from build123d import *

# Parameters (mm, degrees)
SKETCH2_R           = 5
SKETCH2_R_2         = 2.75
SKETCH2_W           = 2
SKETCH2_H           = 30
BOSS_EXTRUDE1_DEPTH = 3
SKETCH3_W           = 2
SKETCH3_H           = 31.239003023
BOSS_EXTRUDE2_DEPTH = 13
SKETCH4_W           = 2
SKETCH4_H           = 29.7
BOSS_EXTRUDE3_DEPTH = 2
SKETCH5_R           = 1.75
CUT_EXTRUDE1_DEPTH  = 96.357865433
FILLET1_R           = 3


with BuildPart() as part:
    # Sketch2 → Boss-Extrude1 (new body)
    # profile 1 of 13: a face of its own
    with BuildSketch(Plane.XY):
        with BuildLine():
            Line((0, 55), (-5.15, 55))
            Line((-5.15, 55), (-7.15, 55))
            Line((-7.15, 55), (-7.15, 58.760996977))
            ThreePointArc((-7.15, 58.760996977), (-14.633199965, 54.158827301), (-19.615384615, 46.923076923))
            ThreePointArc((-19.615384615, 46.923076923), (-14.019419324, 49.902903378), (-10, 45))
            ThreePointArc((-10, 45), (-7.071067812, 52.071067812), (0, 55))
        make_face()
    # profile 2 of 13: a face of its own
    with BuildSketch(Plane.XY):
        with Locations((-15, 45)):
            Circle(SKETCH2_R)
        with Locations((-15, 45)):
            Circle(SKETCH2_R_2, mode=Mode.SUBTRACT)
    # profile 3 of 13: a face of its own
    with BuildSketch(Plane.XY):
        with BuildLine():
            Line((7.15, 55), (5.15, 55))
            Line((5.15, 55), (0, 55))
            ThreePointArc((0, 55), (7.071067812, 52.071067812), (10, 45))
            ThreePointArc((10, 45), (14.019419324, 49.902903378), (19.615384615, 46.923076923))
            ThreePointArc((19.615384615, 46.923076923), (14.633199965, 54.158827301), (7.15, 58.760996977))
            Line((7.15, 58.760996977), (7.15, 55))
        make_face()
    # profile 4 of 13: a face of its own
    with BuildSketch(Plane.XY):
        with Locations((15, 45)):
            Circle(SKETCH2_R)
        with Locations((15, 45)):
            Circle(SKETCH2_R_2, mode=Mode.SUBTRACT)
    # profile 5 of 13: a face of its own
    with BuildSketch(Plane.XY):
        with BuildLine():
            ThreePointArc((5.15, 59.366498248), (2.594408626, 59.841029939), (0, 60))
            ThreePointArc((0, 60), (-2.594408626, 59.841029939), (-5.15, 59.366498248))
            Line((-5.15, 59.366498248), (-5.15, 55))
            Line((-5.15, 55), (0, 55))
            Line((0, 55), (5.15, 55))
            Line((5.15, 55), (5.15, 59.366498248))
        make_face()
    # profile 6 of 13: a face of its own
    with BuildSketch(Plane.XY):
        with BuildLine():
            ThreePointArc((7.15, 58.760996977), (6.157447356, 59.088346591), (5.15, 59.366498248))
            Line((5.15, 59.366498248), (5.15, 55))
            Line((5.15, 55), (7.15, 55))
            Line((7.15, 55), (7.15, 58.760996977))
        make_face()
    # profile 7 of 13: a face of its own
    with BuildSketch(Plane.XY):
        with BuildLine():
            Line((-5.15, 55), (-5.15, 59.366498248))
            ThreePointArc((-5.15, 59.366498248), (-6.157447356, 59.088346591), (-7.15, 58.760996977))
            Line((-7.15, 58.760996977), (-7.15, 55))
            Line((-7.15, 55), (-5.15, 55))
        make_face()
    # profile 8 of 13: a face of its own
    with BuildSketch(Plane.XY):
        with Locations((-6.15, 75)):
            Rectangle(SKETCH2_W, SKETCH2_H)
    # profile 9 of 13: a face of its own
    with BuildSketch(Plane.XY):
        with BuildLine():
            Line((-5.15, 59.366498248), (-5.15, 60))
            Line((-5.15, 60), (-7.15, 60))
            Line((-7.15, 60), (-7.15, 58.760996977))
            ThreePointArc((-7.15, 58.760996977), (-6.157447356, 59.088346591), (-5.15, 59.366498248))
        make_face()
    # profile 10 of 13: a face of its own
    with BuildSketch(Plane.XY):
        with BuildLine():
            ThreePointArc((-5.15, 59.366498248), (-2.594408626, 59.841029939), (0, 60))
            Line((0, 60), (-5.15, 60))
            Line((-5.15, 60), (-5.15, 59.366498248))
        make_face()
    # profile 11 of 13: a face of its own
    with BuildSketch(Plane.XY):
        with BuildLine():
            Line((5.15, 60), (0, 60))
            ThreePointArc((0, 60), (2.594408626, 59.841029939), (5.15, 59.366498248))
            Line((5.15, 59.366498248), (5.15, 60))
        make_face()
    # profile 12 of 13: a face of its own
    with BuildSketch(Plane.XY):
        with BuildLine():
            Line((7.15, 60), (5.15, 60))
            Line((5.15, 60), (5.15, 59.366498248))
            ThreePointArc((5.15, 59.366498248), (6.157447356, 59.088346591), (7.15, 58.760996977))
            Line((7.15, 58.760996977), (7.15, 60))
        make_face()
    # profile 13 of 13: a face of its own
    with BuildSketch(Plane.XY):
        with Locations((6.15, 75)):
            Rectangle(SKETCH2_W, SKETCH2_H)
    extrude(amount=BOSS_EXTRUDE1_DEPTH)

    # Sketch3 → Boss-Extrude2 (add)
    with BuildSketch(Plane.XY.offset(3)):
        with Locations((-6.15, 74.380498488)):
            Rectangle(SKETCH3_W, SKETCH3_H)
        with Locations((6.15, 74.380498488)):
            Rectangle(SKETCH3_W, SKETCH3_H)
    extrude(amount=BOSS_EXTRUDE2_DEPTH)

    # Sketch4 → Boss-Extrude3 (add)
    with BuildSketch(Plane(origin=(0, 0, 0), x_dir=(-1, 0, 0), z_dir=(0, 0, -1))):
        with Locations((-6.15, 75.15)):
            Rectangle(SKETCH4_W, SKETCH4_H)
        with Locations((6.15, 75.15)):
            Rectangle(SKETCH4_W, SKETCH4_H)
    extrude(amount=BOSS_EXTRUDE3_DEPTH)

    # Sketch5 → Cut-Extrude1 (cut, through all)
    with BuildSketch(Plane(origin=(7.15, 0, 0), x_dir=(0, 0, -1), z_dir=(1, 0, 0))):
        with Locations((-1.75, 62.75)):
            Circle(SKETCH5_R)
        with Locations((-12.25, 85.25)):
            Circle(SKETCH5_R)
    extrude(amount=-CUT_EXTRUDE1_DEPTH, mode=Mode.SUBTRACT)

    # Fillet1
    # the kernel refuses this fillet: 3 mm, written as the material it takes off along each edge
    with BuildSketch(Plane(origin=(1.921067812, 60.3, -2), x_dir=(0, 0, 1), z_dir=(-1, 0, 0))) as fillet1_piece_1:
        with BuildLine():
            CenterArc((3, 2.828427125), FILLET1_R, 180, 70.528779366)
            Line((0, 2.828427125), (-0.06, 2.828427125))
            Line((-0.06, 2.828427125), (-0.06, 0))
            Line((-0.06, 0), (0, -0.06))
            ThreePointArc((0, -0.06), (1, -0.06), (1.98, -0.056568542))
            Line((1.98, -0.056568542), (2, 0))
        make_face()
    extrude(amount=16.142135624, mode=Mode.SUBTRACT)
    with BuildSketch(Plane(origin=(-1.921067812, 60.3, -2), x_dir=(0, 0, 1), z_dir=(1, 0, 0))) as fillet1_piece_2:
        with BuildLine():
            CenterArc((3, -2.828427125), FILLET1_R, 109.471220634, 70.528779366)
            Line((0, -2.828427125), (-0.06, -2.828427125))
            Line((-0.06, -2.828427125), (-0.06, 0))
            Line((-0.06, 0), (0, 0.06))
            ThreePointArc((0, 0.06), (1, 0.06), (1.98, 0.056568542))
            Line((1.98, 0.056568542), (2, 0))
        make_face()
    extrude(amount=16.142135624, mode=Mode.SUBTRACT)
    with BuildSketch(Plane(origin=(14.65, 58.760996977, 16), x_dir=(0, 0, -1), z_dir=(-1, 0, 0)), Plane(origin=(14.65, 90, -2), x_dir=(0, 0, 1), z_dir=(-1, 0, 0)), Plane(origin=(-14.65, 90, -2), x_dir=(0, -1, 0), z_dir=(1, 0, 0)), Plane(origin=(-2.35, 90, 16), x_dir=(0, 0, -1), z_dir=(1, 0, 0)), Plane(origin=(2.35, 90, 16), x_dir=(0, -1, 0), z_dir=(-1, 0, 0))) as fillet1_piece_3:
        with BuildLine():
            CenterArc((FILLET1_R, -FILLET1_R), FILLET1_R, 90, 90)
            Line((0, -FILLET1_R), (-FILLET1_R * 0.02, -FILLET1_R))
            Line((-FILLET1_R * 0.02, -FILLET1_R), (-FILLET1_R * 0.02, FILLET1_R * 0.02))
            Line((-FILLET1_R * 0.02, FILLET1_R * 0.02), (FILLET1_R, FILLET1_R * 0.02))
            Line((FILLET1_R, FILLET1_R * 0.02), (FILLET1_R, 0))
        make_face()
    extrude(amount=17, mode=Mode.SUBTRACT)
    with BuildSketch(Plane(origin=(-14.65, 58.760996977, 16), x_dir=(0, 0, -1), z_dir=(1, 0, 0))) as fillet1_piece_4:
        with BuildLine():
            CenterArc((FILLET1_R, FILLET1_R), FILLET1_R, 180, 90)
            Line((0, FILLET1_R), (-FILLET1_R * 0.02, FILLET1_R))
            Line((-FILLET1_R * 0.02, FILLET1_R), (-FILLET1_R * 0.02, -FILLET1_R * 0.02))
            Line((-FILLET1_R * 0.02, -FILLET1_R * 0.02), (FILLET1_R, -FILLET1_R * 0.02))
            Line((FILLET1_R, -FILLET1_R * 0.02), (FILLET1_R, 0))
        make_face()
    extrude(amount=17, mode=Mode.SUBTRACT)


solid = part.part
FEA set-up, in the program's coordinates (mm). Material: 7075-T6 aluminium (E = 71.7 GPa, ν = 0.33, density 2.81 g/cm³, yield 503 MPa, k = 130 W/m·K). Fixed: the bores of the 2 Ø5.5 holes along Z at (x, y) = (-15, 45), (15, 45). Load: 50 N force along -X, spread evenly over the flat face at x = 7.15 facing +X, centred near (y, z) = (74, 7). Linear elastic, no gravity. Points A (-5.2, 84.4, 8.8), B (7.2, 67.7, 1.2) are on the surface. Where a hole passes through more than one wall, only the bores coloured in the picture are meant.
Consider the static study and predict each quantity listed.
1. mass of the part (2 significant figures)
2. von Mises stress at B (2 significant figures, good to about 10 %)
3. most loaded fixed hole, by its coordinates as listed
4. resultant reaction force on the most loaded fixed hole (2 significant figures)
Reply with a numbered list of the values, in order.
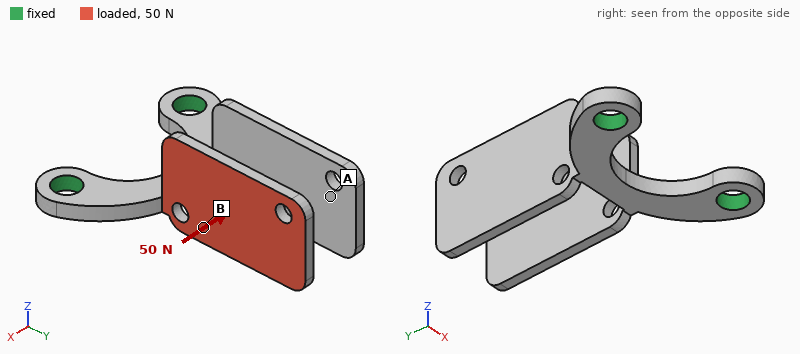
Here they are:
1. 8.7 g
2. 42 MPa
3. (-15, 45)
4. 76 N
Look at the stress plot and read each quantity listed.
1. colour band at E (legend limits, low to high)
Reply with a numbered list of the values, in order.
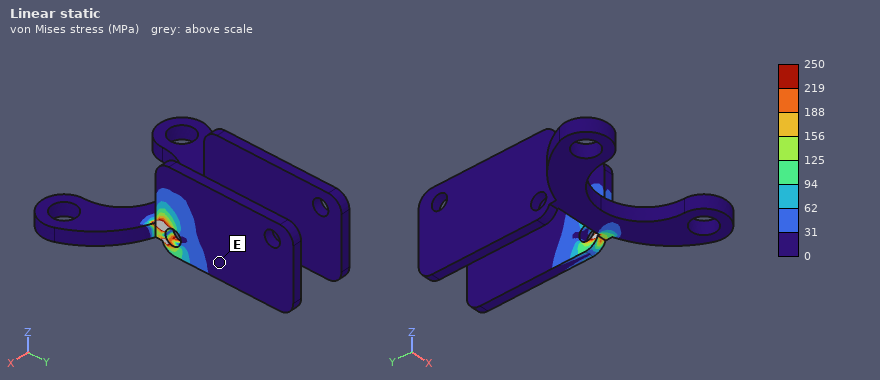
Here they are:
1. 0 to 31 MPa
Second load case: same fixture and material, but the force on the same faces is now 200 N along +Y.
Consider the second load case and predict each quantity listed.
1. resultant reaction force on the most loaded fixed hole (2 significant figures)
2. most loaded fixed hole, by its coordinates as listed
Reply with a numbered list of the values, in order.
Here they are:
1. 180 N
2. (15, 45)
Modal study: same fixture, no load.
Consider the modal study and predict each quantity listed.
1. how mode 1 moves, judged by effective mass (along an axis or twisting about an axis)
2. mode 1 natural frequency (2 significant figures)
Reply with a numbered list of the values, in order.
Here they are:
1. along Z
2. 890 Hz
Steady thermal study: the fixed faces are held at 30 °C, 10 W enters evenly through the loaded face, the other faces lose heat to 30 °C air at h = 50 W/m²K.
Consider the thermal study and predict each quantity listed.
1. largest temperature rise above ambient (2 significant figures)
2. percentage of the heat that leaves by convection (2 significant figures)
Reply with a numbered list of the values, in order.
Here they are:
1. 79 K
2. 35 %
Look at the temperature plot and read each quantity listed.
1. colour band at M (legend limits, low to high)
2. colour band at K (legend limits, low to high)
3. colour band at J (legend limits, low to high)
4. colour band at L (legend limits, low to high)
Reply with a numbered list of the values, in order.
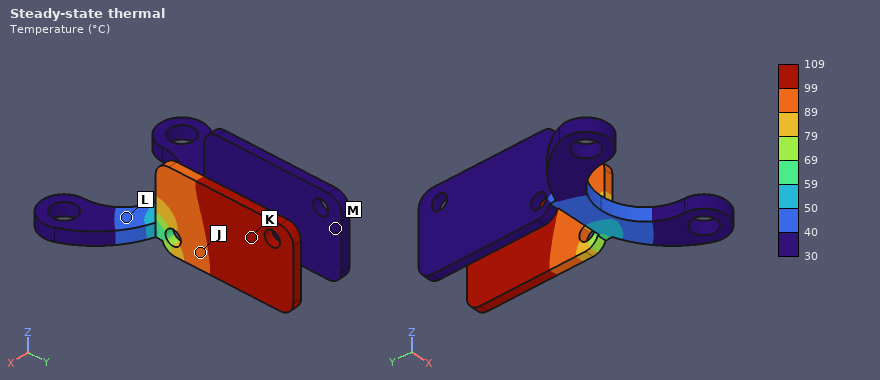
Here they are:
1. 30 to 40 °C
2. 99 to 109 °C
3. 89 to 99 °C
4. 40 to 50 °C
